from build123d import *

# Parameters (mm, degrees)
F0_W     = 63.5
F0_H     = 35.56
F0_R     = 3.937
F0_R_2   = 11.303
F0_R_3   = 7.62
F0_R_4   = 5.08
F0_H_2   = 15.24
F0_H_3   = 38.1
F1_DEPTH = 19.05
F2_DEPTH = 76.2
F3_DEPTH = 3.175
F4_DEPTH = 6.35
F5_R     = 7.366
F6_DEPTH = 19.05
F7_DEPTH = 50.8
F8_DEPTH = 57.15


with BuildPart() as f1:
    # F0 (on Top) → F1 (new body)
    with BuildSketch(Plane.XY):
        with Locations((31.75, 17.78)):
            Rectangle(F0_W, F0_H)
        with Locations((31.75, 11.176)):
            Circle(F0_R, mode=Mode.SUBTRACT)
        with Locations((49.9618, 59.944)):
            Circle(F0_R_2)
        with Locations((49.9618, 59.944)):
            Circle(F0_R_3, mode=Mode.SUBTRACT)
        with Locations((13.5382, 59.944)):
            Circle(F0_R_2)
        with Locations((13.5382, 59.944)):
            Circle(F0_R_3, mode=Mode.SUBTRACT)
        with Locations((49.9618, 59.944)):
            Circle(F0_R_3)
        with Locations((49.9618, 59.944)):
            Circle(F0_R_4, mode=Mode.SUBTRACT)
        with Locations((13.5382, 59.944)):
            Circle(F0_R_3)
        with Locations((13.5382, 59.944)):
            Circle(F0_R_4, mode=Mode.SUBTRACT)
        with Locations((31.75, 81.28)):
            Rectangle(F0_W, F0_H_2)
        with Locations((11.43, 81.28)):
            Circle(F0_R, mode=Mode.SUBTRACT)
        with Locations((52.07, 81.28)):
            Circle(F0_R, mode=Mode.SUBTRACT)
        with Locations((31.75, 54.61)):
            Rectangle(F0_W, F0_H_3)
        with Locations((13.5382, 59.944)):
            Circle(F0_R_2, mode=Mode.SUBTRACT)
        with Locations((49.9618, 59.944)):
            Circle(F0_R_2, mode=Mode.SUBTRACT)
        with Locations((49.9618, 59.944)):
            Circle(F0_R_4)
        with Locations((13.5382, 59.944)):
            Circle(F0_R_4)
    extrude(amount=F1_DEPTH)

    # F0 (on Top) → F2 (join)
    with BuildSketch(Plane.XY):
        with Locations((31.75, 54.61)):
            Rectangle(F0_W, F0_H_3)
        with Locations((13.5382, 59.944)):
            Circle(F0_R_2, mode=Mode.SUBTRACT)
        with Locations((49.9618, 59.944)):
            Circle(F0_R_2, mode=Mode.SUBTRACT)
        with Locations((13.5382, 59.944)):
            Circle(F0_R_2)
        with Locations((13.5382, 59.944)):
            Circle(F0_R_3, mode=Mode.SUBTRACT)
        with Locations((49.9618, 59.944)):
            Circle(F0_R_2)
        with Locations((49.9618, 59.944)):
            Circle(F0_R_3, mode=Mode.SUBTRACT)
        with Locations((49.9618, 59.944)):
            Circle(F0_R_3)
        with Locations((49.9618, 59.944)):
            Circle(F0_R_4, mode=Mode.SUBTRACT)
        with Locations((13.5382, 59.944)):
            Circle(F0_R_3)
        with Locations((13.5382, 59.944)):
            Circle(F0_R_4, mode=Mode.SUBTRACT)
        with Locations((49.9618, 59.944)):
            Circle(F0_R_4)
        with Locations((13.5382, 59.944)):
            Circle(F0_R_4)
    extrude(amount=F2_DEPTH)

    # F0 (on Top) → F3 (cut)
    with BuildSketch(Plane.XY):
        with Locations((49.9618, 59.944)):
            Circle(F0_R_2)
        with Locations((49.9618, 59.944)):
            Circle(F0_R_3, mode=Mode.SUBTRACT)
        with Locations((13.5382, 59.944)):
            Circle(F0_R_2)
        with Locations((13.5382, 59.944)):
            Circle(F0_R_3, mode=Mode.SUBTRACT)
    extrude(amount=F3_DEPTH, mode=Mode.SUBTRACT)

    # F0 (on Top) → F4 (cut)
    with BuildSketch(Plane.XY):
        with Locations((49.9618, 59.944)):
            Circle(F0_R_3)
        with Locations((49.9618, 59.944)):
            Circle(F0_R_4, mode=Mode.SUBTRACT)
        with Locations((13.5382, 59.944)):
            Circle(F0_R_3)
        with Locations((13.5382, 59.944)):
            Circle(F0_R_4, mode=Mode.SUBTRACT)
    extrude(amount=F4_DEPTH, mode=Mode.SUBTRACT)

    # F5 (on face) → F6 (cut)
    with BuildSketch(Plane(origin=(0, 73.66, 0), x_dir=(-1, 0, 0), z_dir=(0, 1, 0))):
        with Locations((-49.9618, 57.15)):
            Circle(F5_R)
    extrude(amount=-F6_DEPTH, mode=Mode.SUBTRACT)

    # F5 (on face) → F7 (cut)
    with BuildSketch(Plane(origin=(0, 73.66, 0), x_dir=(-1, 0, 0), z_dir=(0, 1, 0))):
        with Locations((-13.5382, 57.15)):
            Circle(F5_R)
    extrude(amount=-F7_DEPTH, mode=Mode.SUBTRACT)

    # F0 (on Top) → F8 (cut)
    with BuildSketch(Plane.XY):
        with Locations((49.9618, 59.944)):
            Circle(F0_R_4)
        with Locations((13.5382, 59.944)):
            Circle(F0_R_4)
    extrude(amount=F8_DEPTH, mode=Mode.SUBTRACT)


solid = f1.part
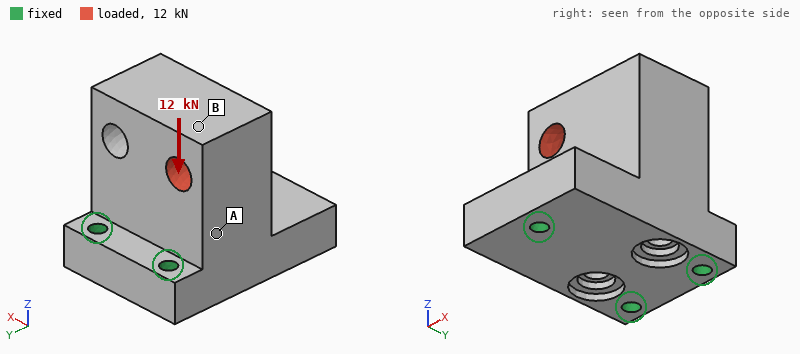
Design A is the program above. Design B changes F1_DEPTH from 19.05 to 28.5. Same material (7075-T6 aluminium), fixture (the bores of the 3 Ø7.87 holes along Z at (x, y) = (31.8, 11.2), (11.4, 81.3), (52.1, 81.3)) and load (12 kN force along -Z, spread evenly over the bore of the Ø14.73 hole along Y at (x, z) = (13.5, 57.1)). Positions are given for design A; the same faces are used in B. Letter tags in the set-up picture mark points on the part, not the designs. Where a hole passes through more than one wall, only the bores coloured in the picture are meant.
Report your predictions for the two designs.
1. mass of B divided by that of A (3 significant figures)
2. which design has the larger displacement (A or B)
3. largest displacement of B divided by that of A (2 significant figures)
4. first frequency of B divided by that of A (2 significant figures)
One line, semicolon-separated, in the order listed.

1.13; A; 0.59; 1.4
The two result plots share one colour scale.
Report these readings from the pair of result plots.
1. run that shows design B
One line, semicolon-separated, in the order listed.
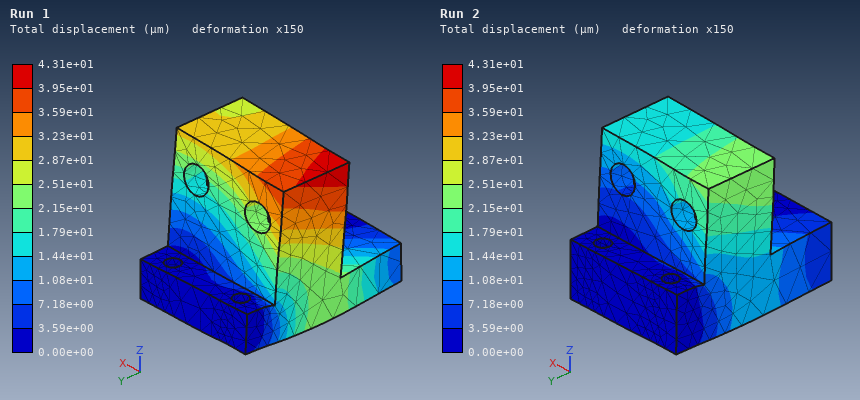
Run 2
